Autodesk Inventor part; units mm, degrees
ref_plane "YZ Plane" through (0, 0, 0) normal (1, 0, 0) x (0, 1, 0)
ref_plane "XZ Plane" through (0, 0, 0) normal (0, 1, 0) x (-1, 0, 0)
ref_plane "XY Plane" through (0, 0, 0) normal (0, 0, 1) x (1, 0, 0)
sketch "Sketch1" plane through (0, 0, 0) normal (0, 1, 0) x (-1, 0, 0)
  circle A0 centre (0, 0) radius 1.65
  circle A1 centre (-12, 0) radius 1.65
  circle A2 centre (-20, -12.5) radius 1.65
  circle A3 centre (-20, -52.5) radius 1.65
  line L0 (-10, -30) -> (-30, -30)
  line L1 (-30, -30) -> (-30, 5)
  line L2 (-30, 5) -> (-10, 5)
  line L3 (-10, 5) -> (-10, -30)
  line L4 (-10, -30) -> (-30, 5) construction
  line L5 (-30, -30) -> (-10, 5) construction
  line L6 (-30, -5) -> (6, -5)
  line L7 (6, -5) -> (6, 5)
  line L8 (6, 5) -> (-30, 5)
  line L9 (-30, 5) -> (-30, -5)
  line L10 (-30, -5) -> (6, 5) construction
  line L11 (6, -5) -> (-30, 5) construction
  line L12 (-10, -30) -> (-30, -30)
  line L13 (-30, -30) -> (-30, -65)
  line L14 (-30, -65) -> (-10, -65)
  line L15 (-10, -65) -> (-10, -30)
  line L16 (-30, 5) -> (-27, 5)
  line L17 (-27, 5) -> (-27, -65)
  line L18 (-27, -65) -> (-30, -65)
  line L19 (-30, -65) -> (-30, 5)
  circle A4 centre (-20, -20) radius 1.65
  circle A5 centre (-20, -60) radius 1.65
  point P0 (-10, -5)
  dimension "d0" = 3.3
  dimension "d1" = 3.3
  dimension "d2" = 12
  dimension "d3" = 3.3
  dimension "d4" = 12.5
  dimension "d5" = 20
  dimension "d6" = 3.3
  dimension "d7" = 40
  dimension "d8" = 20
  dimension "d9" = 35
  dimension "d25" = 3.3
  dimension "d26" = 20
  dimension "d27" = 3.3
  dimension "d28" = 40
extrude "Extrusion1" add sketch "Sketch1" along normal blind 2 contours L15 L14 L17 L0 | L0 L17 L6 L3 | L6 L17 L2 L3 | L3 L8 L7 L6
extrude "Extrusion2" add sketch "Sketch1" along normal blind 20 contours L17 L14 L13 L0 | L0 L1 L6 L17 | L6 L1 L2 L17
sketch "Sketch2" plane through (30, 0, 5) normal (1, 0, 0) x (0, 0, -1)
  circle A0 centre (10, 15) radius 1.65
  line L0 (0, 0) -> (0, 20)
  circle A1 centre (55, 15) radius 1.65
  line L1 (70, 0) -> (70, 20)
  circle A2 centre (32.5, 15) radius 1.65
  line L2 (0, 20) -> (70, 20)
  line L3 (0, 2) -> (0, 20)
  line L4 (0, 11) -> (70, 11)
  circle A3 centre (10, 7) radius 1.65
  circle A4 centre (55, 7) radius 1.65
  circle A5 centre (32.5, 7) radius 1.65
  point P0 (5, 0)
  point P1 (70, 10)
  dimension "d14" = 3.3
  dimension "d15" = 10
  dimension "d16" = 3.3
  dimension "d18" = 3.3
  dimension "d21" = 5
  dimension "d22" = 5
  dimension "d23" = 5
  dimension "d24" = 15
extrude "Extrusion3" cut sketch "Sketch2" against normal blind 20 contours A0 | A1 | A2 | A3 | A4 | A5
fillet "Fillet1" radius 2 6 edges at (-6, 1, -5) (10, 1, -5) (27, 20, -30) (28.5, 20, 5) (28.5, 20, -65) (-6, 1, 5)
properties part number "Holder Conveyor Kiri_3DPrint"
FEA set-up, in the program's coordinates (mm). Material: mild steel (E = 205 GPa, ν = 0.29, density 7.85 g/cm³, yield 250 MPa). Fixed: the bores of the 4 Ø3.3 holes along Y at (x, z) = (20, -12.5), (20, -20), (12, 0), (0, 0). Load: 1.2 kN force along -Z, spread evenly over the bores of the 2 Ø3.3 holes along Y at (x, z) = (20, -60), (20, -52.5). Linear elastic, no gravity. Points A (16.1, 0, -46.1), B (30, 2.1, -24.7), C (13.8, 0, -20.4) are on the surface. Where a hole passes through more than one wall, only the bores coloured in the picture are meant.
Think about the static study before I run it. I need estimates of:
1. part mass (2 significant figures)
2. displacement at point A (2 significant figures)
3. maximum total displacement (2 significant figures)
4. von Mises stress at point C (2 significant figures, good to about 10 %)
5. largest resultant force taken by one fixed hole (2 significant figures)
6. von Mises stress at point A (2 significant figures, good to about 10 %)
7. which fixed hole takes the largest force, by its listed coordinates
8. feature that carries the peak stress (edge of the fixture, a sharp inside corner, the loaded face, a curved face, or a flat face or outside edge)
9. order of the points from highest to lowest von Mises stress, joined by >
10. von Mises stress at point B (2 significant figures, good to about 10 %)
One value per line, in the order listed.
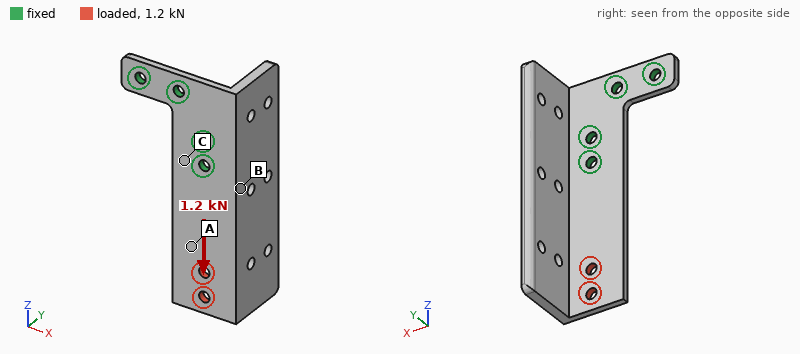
52 g
5.4 µm
9.6 µm
22 MPa
800 N
35 MPa
(20, -20)
the loaded face
A > C > B
9.2 MPa
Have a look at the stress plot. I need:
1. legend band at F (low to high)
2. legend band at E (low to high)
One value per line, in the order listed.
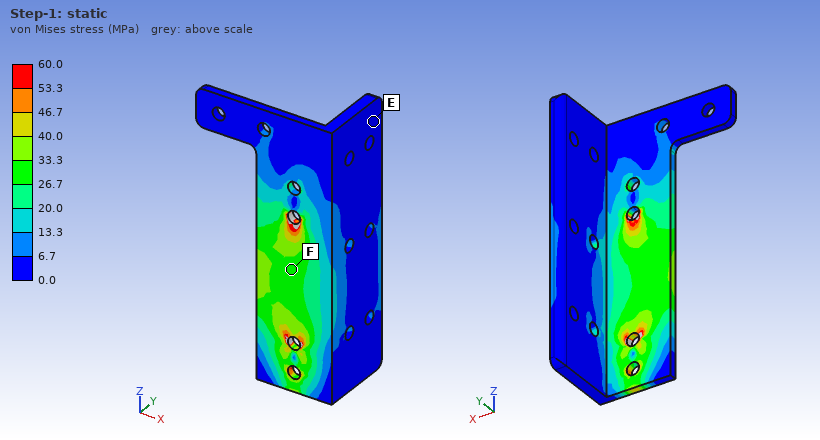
26.7 to 33.3 MPa
0.0 to 6.7 MPa
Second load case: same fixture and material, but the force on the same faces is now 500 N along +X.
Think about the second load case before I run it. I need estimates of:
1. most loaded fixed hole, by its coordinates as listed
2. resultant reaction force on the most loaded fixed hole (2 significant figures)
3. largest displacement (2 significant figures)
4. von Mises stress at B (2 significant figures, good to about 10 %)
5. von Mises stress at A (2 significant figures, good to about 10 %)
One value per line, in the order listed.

(20, -20)
1.4 kN
64 µm
70 MPa
27 MPa
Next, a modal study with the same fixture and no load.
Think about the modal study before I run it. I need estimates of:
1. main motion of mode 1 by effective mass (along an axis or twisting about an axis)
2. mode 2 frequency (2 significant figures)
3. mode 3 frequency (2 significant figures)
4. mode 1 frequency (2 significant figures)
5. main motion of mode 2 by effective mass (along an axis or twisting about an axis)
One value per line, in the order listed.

along Y
1800 Hz
3700 Hz
1500 Hz
along X
